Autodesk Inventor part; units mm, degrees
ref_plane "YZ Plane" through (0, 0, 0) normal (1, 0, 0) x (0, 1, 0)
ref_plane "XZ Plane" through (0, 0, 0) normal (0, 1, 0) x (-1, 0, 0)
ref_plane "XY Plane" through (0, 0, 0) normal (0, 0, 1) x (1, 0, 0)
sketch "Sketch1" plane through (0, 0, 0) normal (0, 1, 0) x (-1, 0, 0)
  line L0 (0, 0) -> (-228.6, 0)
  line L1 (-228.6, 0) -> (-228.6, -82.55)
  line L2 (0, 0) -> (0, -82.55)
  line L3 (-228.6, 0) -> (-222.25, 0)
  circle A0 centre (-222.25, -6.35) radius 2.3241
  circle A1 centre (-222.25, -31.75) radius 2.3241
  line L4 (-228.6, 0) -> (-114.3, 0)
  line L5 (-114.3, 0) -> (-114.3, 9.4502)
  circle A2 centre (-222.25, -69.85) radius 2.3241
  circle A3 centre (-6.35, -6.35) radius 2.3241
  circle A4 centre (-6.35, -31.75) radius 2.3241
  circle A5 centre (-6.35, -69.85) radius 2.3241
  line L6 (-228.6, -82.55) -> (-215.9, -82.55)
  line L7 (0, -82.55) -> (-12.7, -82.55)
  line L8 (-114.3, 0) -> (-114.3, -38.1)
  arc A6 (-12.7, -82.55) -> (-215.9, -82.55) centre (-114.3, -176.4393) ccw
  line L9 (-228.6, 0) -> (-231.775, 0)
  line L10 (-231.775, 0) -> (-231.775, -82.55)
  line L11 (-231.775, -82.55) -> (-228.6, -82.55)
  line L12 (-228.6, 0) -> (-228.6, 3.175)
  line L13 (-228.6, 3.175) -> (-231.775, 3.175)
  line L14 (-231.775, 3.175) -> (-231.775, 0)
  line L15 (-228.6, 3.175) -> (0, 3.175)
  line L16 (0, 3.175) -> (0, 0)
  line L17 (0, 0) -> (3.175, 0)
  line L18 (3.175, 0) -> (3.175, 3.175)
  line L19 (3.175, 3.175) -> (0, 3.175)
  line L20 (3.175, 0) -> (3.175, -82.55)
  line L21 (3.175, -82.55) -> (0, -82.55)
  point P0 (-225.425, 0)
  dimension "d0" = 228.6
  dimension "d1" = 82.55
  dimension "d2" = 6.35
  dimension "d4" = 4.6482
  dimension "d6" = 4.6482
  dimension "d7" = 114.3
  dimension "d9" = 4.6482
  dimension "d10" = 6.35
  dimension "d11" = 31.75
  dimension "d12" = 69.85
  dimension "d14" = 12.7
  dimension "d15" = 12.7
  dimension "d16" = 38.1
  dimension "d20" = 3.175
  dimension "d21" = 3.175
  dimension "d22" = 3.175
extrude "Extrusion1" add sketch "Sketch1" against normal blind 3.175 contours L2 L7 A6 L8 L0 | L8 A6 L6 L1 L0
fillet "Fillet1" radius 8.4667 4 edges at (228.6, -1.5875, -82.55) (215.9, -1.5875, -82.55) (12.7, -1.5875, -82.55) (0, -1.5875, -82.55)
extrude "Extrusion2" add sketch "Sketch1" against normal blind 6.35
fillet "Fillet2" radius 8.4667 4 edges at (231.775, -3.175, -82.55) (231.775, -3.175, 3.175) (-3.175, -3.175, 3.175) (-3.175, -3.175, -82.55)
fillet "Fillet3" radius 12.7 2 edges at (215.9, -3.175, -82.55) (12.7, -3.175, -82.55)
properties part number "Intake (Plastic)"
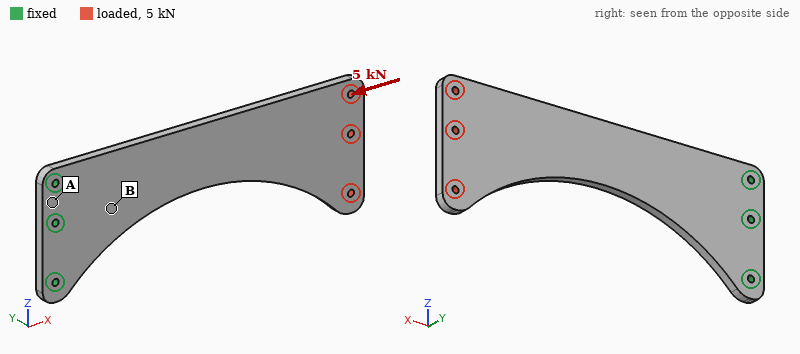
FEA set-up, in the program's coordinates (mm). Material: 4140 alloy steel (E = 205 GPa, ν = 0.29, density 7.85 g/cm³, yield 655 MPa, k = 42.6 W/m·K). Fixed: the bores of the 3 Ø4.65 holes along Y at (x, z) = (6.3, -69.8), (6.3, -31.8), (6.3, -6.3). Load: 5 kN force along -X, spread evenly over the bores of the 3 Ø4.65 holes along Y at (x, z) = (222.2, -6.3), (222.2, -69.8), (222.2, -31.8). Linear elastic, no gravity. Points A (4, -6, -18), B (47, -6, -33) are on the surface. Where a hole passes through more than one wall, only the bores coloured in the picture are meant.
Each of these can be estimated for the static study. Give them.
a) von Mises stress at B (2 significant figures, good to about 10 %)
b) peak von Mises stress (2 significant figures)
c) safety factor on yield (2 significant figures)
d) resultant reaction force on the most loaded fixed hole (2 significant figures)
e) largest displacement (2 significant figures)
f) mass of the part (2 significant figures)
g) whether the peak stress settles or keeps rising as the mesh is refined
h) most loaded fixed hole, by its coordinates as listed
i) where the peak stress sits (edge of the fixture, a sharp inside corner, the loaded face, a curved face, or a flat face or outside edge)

20 MPa
75 MPa
8.7
2.2 kN
0.17 mm
680 g
settles
(6.3, -31.8)
a curved face
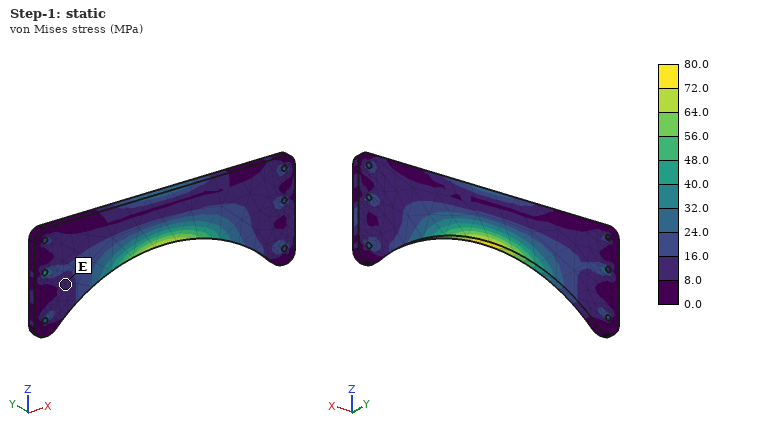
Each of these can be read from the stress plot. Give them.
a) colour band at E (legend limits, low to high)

8.0 to 16.0 MPa
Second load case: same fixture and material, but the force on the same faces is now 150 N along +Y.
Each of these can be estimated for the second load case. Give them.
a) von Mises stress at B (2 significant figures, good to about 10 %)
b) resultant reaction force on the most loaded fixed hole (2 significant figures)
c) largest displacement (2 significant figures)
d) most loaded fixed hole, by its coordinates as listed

66 MPa
240 N
2.3 mm
(6.3, -31.8)
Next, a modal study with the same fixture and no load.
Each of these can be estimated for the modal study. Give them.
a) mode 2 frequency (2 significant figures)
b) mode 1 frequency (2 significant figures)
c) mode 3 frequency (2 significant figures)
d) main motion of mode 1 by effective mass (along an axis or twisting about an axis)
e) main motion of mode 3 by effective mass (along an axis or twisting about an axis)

530 Hz
94 Hz
740 Hz
along Y
along Z
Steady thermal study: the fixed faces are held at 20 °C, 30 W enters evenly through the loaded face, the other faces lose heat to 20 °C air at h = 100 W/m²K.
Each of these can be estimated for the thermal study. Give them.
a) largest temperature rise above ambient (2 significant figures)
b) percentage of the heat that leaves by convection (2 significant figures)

47 K
100 %
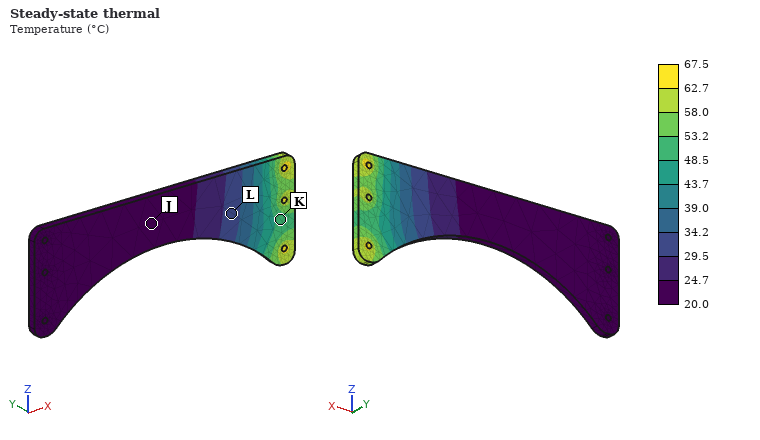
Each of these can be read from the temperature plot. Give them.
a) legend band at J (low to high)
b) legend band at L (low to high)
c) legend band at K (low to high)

20.0 to 24.7 °C
29.5 to 34.2 °C
48.5 to 53.2 °C
